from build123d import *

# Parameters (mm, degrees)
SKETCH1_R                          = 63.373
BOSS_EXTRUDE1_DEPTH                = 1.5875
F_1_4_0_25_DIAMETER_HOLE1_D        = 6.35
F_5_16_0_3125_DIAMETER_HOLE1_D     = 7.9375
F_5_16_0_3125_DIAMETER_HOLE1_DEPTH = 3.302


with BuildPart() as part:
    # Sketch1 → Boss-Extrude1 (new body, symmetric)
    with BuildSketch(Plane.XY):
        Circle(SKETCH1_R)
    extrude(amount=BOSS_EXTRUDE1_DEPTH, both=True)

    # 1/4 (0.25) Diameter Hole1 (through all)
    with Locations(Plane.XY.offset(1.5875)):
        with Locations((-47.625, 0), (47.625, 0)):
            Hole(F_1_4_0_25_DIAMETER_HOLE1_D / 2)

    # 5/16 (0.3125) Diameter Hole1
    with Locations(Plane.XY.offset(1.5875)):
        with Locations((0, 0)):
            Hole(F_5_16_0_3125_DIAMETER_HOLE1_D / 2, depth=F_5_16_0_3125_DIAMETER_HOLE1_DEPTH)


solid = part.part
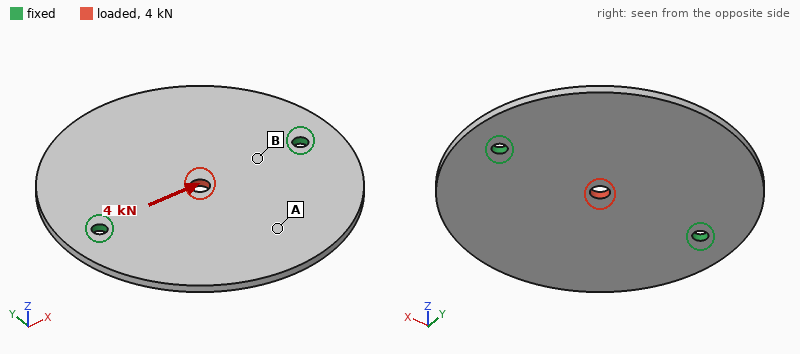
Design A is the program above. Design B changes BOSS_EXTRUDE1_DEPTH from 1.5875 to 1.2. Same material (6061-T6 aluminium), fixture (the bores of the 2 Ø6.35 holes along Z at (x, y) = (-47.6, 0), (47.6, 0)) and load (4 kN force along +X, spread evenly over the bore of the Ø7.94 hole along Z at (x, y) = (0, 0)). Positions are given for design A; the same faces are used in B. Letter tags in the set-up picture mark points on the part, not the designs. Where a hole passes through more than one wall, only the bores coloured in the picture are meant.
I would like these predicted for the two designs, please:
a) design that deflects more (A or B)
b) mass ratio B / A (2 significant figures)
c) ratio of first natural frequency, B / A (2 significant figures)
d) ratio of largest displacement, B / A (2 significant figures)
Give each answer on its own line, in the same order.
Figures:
B
0.76
0.77
1.3
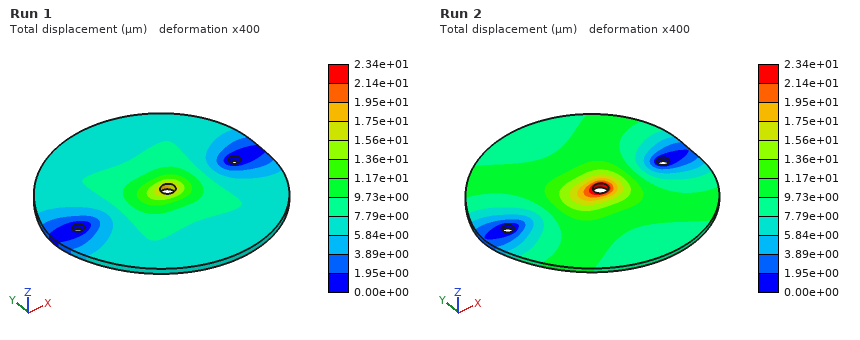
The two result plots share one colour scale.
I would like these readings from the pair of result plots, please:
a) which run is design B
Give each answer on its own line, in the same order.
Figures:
Run 2
